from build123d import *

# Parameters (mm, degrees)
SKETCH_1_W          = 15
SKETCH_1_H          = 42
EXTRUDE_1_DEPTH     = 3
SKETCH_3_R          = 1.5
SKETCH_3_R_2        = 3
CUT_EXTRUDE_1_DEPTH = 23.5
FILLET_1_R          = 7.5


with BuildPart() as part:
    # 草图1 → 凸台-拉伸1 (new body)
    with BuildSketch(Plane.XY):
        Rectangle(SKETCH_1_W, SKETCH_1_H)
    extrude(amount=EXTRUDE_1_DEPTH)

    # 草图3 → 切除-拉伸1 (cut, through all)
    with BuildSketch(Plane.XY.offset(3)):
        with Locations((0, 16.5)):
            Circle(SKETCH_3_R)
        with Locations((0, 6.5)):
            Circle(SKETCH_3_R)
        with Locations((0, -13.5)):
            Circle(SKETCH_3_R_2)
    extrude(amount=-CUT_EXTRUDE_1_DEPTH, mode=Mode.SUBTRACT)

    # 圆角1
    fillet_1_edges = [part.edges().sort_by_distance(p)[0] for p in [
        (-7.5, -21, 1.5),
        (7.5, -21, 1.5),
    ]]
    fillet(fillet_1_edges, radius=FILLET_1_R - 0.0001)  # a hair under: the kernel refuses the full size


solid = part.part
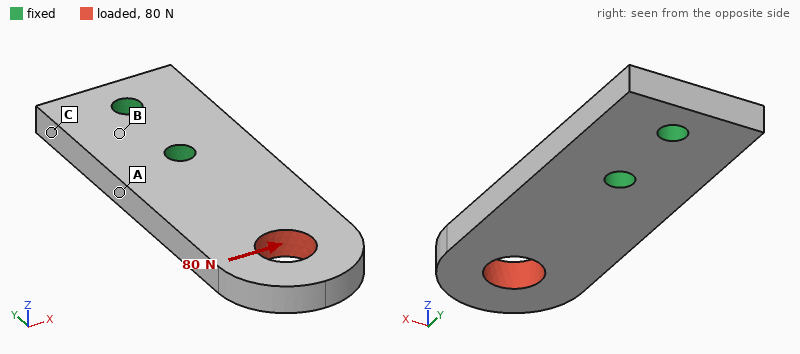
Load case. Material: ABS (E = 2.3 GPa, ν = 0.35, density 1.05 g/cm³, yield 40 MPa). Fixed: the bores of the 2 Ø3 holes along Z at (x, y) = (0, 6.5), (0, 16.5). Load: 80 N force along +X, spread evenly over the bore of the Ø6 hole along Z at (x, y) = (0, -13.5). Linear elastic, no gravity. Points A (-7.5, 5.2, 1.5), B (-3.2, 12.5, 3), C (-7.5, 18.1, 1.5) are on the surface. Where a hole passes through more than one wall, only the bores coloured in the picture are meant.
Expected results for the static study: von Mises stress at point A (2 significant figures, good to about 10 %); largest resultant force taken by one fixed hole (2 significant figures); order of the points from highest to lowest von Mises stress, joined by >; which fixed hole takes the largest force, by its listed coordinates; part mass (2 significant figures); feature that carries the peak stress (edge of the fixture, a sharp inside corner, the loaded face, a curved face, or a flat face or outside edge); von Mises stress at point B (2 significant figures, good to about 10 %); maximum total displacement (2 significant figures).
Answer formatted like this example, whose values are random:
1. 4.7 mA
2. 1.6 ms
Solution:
1. 14 MPa
2. 190 N
3. A > B > C
4. (0, 6.5)
5. 1.8 g
6. edge of the fixture
7. 5.9 MPa
8. 0.39 mm
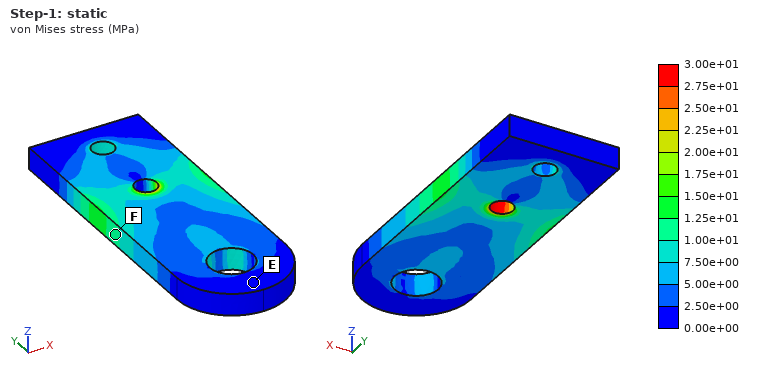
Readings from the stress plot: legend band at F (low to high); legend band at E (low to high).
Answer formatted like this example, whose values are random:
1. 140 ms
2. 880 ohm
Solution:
1. 1.00e+01 to 1.25e+01 MPa
2. 0.00e+00 to 2.50e+00 MPa
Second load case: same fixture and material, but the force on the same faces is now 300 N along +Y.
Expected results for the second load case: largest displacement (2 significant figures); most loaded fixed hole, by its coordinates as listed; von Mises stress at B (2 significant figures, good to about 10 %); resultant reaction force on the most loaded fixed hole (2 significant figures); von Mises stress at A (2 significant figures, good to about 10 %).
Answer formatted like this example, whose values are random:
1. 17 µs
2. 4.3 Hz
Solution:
1. 99 µm
2. (0, 6.5)
3. 2.4 MPa
4. 240 N
5. 3.9 MPa
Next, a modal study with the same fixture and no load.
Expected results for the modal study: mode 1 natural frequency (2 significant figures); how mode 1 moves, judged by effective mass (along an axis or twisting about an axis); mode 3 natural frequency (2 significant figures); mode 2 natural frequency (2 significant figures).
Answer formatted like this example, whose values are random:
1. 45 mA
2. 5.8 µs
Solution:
1. 1100 Hz
2. along Z
3. 3400 Hz
4. 3400 Hz
